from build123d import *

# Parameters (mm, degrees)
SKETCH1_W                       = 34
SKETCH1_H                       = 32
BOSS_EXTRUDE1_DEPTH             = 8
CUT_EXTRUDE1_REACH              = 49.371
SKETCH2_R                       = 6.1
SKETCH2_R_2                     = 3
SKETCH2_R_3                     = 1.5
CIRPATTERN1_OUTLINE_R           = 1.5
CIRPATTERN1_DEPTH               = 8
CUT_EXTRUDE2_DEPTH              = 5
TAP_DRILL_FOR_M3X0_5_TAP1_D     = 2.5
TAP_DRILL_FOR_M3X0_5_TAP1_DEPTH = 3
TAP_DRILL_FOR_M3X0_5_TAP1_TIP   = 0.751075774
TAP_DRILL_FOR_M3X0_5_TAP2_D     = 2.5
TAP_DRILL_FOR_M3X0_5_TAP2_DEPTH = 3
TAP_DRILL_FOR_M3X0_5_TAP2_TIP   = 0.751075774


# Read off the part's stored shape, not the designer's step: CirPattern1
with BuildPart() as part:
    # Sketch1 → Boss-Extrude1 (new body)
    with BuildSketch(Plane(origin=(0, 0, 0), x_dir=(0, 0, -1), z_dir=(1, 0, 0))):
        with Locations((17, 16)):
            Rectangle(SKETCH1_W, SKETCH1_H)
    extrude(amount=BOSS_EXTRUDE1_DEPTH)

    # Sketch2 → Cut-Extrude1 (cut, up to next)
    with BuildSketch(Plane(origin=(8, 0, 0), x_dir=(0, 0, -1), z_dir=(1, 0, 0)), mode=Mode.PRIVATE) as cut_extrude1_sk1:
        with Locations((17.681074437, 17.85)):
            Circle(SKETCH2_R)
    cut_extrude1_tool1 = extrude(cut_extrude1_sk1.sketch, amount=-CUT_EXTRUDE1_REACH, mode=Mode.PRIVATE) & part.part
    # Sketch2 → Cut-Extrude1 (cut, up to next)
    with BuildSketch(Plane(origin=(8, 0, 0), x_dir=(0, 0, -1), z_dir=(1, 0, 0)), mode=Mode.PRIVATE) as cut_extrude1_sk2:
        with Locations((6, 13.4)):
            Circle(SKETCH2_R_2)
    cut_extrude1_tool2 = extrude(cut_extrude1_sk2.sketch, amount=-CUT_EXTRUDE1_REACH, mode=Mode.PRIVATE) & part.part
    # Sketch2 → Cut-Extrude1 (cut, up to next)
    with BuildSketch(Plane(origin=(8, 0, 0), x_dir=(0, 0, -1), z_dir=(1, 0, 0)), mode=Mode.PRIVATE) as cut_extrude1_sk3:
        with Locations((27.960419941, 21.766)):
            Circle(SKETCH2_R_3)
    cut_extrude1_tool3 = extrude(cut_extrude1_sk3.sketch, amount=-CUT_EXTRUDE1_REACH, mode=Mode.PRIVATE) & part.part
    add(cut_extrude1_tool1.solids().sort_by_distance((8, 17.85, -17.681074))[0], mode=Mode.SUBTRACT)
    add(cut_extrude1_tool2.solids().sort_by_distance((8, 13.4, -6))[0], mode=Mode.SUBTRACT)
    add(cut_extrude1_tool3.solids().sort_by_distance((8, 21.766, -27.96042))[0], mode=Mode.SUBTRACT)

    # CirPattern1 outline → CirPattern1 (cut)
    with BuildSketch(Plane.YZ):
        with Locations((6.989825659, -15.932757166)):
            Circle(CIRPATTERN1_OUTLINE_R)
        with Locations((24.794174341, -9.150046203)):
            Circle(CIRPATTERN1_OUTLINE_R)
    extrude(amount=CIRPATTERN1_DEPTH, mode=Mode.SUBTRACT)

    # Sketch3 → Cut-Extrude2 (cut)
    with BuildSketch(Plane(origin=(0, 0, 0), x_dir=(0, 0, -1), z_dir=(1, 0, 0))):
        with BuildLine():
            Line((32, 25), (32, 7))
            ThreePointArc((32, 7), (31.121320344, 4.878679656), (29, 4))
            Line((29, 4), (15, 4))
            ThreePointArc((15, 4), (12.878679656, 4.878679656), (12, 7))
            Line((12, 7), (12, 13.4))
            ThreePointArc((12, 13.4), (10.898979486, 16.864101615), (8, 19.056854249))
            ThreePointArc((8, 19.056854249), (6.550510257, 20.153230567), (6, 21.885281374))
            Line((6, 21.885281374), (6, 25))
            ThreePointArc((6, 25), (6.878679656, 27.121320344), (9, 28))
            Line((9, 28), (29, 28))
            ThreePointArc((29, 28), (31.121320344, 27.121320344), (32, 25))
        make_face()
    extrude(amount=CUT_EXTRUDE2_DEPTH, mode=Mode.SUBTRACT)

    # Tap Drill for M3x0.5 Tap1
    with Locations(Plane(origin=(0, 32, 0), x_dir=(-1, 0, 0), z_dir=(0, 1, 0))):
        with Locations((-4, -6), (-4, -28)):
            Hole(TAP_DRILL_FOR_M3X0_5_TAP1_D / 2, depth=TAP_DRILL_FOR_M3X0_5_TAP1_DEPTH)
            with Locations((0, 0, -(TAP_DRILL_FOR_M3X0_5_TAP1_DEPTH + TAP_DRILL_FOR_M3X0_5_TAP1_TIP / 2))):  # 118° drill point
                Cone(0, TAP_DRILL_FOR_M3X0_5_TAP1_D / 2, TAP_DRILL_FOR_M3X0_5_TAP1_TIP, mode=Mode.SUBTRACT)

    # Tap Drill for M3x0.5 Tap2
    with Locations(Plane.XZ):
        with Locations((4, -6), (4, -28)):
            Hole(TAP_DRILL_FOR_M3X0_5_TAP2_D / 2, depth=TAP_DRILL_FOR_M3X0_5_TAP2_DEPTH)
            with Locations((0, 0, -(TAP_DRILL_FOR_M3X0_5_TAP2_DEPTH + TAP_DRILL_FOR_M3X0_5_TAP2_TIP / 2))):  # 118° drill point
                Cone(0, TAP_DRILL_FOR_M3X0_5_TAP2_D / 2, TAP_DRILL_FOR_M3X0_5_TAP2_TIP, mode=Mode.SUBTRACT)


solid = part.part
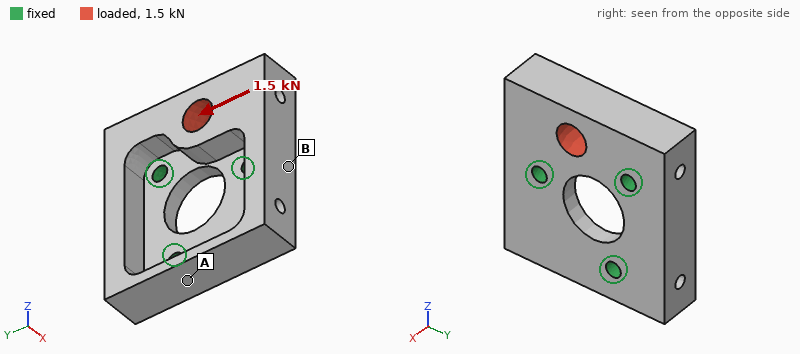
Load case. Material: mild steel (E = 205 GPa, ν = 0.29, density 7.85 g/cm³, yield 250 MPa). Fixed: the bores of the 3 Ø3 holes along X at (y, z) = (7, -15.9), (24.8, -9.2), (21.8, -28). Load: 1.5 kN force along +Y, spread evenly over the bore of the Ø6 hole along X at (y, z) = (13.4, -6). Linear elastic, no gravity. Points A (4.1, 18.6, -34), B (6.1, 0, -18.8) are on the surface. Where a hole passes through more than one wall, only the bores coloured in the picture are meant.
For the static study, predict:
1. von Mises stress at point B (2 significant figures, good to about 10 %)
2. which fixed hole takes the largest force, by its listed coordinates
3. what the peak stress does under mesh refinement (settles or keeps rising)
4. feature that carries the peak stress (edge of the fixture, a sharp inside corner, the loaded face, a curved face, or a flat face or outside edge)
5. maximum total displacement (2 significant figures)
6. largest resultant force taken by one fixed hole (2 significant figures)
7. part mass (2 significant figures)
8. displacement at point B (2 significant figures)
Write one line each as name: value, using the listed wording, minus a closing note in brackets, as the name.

von Mises stress at point B: 14 MPa
which fixed hole takes the largest force, by its listed coordinates: (24.8, -9.2)
what the peak stress does under mesh refinement: keeps rising
feature that carries the peak stress: edge of the fixture
maximum total displacement: 5.0 µm
largest resultant force taken by one fixed hole: 1.1 kN
part mass: 42 g
displacement at point B: 0.87 µm
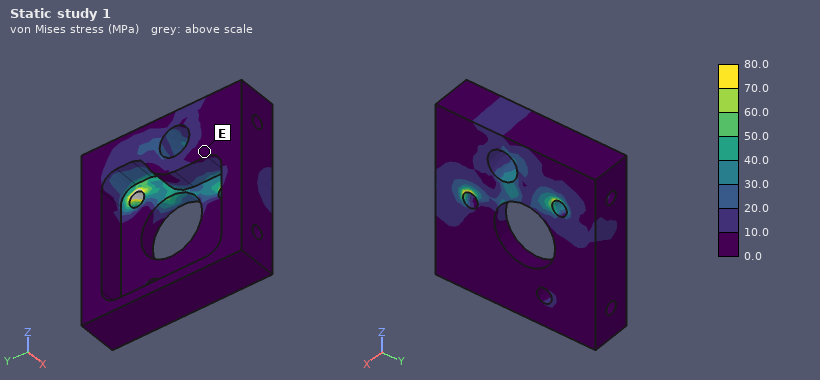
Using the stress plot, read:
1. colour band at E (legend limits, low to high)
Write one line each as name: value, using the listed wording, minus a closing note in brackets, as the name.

colour band at E: 0.0 to 10.0 MPa
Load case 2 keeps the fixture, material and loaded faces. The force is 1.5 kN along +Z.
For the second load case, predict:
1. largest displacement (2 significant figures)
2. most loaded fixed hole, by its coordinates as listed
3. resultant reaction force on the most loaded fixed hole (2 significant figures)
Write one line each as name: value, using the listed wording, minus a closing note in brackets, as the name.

largest displacement: 9.0 µm
most loaded fixed hole, by its coordinates as listed: (7, -15.9)
resultant reaction force on the most loaded fixed hole: 1.0 kN
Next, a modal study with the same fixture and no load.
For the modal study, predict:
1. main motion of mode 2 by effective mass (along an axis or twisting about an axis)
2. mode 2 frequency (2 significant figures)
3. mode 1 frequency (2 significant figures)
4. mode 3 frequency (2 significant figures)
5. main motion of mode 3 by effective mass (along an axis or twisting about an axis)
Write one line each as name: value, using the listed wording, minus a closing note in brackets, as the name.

main motion of mode 2 by effective mass: along X
mode 2 frequency: 14 kHz
mode 1 frequency: 9900 Hz
mode 3 frequency: 21 kHz
main motion of mode 3 by effective mass: along X
